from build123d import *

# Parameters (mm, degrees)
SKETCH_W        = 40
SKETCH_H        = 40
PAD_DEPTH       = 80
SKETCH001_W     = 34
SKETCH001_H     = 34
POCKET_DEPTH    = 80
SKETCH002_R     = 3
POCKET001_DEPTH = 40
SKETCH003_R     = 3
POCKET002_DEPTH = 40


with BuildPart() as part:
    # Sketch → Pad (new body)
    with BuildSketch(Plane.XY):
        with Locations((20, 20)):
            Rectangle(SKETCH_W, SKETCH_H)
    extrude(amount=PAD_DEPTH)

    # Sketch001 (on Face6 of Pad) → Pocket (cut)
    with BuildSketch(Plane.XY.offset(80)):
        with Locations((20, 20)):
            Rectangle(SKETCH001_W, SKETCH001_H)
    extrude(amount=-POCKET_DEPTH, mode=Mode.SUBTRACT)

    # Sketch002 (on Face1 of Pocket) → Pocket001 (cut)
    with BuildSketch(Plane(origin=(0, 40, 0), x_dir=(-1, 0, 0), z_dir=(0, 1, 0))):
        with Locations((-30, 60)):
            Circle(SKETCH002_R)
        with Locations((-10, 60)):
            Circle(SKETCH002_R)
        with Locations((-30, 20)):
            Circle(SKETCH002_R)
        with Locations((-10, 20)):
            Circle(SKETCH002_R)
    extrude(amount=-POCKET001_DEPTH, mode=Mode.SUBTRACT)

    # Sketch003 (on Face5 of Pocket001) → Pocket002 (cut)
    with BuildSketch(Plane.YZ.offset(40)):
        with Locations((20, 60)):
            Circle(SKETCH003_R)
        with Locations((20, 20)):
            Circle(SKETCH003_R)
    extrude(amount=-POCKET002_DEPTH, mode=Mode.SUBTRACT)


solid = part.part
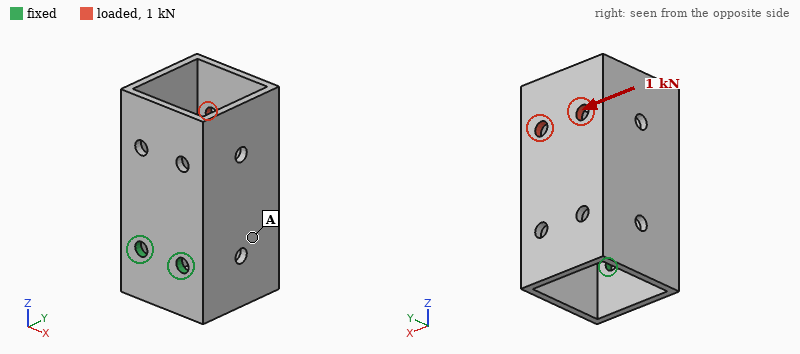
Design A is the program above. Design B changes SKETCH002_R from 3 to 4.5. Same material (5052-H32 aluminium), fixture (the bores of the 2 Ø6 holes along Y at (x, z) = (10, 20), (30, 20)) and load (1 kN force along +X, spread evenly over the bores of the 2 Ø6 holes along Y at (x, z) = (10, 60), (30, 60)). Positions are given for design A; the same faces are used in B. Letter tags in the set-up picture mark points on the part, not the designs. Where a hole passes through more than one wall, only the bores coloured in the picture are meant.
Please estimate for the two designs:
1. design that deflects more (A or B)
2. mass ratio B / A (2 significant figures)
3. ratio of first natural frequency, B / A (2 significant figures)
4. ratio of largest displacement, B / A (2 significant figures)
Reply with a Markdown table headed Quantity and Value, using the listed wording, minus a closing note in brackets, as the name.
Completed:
| Quantity | Value |
|---|---|
| design that deflects more | A |
| mass ratio B / A | 0.98 |
| ratio of first natural frequency, B / A | 1.3 |
| ratio of largest displacement, B / A | 0.91 |
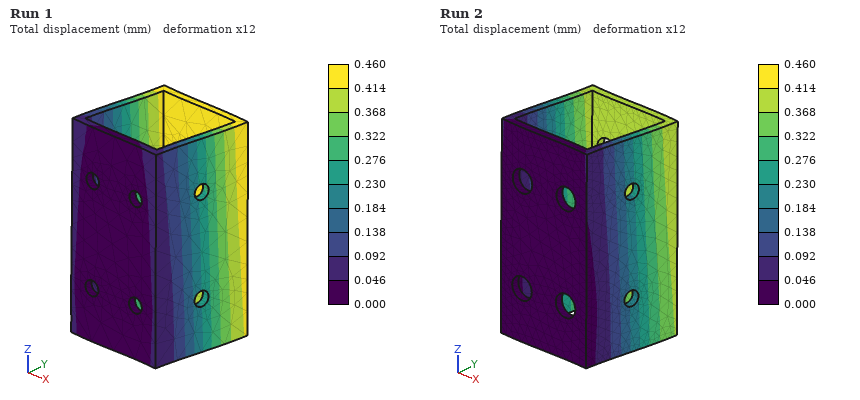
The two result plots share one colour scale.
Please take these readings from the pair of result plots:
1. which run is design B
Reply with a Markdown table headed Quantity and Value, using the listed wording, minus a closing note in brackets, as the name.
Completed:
| Quantity | Value |
|---|---|
| which run is design B | Run 2 |
